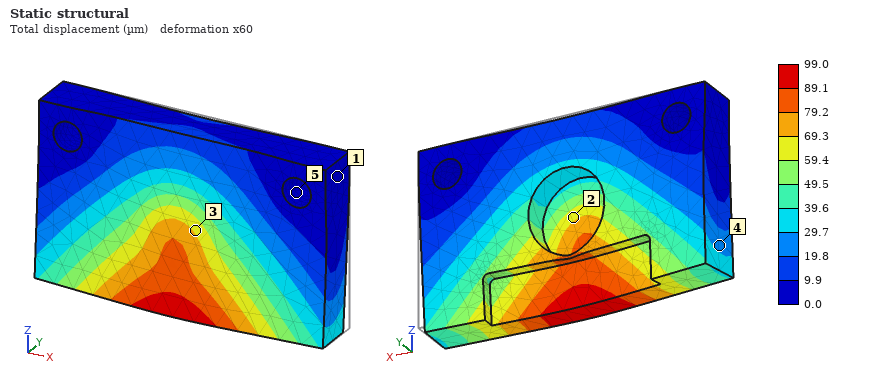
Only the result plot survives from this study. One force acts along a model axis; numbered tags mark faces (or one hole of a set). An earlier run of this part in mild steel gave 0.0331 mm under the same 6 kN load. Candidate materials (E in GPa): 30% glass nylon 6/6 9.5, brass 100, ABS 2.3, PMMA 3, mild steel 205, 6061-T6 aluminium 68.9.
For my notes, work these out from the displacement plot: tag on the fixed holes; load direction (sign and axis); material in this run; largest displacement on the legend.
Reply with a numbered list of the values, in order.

1. 5
2. -Y
3. 6061-T6 aluminium
4. 99.0 µm
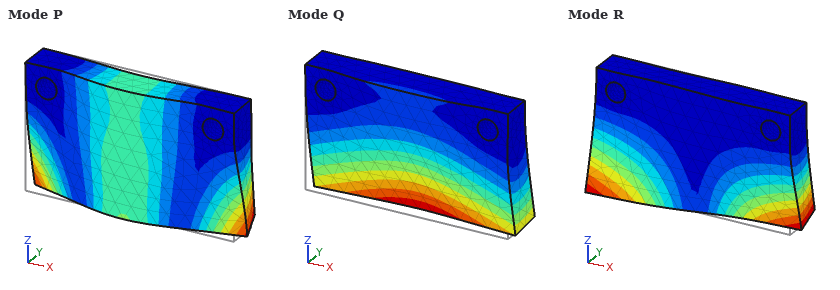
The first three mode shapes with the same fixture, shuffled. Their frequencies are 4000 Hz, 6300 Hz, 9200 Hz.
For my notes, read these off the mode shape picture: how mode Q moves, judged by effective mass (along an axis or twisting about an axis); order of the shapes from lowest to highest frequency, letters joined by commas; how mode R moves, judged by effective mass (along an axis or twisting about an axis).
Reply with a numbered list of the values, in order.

1. along Y
2. Q, R, P
3. twisting about Z
